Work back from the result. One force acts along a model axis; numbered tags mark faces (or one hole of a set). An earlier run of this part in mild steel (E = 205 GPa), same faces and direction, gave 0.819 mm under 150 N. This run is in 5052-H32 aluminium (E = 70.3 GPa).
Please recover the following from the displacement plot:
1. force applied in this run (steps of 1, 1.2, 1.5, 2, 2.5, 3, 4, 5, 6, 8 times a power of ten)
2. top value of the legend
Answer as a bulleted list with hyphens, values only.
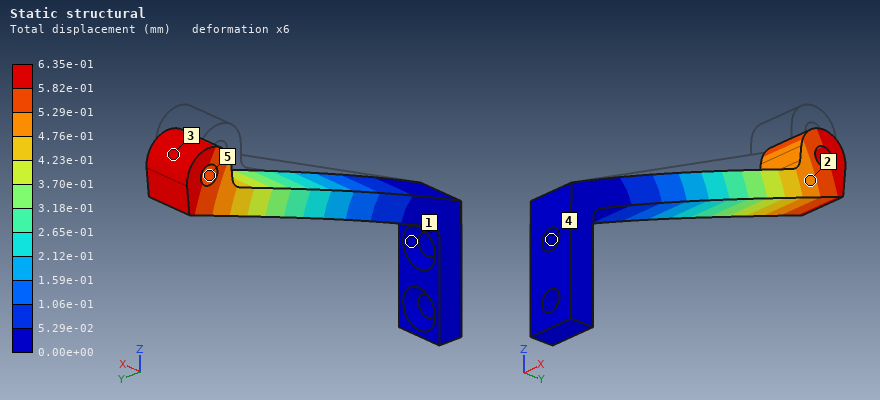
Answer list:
- 40 N
- 6.35e-01 mm
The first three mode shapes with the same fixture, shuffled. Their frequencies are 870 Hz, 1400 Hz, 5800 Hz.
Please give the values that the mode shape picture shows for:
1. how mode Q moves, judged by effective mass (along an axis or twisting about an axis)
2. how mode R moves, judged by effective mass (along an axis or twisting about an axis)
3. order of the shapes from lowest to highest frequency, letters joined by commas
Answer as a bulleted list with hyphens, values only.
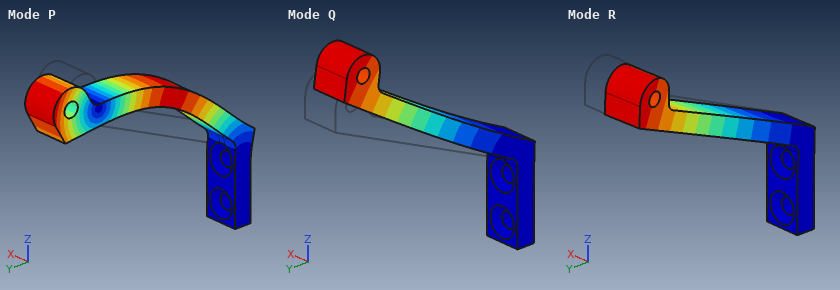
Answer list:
- along Z
- along X
- Q, R, P
